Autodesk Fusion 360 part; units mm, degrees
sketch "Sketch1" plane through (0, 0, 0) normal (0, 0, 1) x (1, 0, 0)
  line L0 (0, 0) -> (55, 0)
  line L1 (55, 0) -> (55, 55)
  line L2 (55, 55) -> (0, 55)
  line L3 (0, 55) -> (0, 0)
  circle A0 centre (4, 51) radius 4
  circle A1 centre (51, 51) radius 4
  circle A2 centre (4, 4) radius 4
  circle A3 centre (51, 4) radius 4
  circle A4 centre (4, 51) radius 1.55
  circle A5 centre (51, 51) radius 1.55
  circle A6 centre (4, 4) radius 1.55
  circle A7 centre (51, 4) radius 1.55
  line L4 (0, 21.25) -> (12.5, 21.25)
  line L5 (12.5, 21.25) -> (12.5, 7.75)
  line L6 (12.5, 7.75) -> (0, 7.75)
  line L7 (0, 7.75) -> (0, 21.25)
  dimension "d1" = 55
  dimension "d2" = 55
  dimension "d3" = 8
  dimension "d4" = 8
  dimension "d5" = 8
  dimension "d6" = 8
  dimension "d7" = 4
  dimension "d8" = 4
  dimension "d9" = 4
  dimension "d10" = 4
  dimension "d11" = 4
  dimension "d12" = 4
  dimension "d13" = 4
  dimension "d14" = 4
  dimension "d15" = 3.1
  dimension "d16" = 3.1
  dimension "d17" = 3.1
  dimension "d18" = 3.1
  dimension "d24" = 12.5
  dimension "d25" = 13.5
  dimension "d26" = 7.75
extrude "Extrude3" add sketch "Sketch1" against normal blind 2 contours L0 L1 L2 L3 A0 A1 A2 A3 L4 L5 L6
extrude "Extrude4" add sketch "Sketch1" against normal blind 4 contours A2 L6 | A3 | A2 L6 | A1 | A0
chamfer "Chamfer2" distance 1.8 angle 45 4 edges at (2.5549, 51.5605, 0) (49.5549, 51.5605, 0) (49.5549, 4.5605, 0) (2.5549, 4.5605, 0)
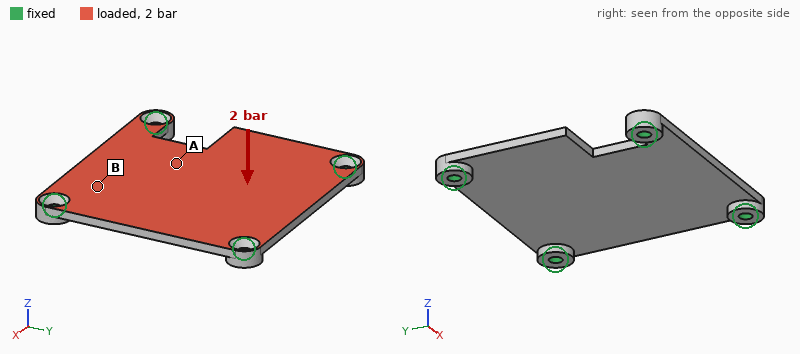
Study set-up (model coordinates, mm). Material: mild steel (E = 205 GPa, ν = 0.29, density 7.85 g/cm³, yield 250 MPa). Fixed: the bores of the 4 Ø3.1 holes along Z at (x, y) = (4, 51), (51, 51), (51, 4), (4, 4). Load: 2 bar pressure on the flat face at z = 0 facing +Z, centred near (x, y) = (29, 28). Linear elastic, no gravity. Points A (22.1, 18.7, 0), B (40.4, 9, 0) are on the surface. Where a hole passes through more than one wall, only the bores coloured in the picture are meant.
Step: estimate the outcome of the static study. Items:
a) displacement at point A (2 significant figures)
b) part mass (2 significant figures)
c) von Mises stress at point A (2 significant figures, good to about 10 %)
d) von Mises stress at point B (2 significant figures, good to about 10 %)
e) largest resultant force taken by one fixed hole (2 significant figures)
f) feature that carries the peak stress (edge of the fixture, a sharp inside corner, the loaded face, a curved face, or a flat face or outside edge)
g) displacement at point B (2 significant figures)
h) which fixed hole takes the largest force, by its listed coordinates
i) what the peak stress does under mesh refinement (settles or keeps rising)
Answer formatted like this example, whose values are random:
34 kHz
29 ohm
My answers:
44 µm
46 g
34 MPa
15 MPa
300 N
edge of the fixture
16 µm
(51, 4)
keeps rising
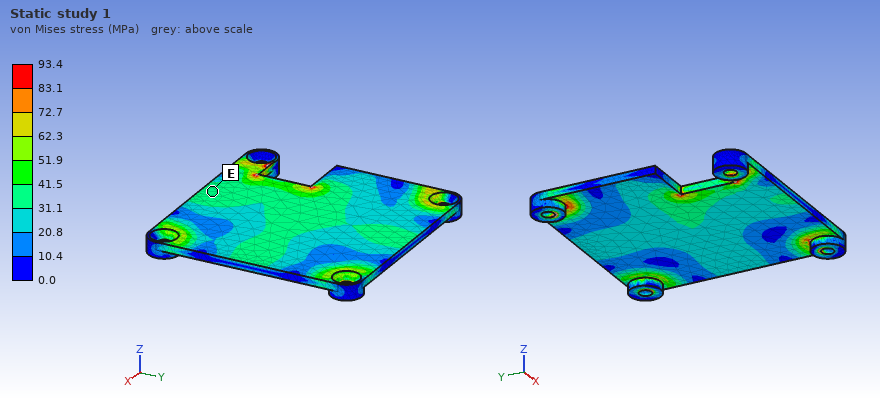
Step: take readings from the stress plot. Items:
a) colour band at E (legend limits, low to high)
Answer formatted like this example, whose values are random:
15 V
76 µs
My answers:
31.1 to 41.5 MPa
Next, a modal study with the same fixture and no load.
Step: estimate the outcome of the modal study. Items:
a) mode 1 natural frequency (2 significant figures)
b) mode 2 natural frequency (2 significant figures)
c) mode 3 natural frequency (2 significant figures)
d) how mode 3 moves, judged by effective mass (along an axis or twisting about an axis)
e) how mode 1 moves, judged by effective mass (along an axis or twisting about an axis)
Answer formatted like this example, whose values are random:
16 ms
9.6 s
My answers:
3100 Hz
4800 Hz
5700 Hz
twisting about X
along Z
